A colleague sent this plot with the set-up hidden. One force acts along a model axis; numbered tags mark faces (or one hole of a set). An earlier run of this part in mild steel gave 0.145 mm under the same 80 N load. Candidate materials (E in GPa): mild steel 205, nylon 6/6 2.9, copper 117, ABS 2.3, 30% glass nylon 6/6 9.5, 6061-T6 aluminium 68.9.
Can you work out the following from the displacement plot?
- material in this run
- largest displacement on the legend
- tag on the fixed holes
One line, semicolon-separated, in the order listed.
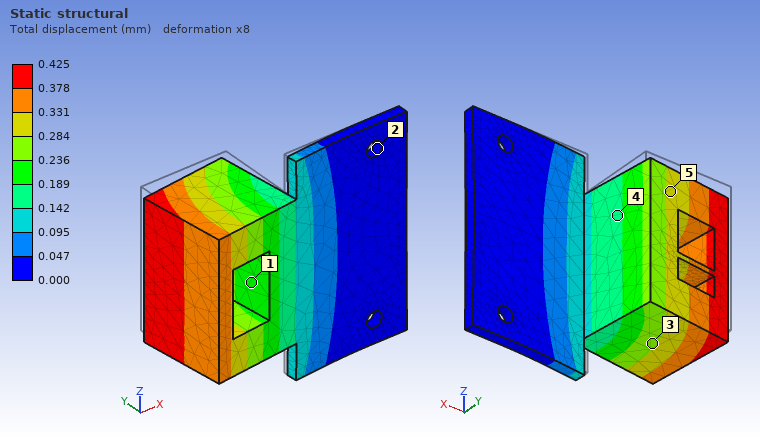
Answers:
6061-T6 aluminium; 0.425 mm; 2
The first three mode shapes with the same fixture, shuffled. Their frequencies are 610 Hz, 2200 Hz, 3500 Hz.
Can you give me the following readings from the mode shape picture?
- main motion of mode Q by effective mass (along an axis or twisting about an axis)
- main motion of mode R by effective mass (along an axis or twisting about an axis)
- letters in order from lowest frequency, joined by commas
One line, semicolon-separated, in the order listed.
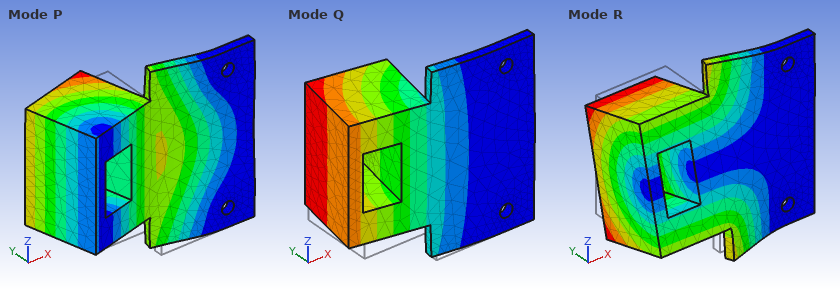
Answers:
along Y; along Z; Q, R, P
